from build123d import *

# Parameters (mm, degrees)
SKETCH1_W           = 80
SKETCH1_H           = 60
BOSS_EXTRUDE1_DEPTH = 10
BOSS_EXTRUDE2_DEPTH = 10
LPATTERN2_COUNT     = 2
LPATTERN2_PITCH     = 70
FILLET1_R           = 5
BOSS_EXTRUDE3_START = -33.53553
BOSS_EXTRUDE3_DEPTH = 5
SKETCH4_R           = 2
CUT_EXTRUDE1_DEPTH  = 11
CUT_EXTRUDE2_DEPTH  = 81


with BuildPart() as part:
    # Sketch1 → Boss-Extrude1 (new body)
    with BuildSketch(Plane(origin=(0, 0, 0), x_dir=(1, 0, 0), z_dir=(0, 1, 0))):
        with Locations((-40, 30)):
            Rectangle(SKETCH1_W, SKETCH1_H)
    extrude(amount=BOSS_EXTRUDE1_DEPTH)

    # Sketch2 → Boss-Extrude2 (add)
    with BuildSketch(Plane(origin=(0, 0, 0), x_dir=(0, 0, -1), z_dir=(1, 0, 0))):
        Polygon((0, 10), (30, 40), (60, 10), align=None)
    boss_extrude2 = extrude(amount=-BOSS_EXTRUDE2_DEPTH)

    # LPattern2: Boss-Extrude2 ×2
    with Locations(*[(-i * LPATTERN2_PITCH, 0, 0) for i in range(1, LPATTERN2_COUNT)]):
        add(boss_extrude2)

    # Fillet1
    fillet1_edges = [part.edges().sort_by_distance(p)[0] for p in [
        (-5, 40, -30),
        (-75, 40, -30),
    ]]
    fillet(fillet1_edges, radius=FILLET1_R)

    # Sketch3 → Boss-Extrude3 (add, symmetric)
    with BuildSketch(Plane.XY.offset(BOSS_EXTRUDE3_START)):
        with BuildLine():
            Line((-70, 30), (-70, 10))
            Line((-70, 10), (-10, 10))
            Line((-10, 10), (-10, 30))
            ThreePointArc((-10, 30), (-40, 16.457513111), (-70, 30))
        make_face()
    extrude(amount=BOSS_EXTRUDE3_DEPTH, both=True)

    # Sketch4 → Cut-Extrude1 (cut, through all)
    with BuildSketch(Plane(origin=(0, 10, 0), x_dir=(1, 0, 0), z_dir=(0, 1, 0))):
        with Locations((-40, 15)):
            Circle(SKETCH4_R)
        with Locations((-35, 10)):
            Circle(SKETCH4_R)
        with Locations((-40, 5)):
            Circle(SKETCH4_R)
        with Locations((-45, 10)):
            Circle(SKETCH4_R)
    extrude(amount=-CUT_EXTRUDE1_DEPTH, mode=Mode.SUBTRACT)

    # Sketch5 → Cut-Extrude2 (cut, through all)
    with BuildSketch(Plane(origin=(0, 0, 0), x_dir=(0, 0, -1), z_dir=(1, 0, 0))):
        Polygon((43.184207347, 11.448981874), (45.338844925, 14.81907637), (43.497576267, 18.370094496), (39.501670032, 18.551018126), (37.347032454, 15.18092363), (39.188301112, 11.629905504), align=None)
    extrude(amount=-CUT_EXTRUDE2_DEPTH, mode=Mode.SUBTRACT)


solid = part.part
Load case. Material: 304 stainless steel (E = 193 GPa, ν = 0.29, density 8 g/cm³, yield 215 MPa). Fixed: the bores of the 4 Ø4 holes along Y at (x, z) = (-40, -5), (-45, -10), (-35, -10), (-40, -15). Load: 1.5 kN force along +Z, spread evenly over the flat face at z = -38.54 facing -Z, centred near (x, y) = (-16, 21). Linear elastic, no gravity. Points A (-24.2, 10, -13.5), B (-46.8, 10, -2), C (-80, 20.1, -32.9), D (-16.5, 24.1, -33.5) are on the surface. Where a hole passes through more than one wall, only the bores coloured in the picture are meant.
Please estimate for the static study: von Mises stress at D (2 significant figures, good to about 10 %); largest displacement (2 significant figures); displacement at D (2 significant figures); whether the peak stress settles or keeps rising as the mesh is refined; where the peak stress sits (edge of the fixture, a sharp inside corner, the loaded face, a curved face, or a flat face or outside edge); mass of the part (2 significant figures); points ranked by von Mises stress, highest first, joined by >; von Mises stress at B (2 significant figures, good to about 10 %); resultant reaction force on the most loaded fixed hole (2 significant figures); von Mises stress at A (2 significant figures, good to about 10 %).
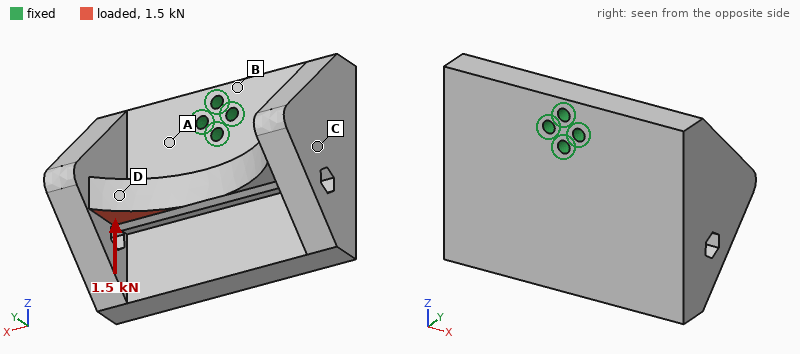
9.6 MPa
27 µm
18 µm
keeps rising
edge of the fixture
570 g
A > B > D > C
17 MPa
1.9 kN
28 MPa
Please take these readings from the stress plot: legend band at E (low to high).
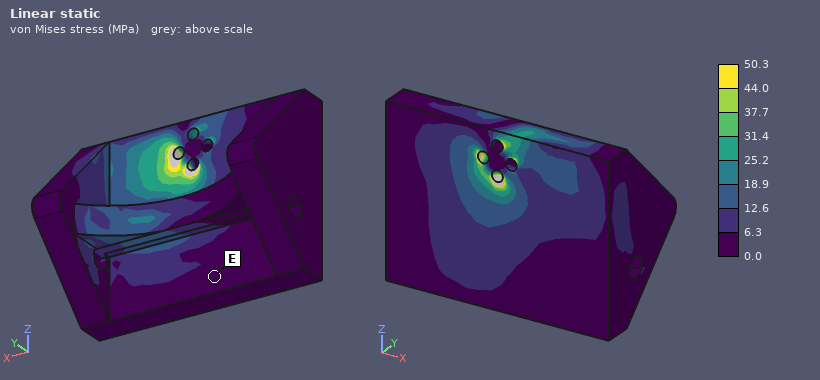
0.0 to 6.3 MPa
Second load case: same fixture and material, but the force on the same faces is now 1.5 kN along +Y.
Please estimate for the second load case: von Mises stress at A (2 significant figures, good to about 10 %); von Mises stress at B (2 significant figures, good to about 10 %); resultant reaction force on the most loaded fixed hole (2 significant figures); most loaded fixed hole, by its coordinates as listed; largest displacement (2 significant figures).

32 MPa
21 MPa
1.8 kN
(-40, -15)
51 µm
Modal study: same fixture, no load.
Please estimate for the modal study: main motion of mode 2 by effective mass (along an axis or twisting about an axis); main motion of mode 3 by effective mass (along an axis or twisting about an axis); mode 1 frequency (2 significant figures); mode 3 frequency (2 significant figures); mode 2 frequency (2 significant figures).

along Y
along X
2200 Hz
3200 Hz
2300 Hz
